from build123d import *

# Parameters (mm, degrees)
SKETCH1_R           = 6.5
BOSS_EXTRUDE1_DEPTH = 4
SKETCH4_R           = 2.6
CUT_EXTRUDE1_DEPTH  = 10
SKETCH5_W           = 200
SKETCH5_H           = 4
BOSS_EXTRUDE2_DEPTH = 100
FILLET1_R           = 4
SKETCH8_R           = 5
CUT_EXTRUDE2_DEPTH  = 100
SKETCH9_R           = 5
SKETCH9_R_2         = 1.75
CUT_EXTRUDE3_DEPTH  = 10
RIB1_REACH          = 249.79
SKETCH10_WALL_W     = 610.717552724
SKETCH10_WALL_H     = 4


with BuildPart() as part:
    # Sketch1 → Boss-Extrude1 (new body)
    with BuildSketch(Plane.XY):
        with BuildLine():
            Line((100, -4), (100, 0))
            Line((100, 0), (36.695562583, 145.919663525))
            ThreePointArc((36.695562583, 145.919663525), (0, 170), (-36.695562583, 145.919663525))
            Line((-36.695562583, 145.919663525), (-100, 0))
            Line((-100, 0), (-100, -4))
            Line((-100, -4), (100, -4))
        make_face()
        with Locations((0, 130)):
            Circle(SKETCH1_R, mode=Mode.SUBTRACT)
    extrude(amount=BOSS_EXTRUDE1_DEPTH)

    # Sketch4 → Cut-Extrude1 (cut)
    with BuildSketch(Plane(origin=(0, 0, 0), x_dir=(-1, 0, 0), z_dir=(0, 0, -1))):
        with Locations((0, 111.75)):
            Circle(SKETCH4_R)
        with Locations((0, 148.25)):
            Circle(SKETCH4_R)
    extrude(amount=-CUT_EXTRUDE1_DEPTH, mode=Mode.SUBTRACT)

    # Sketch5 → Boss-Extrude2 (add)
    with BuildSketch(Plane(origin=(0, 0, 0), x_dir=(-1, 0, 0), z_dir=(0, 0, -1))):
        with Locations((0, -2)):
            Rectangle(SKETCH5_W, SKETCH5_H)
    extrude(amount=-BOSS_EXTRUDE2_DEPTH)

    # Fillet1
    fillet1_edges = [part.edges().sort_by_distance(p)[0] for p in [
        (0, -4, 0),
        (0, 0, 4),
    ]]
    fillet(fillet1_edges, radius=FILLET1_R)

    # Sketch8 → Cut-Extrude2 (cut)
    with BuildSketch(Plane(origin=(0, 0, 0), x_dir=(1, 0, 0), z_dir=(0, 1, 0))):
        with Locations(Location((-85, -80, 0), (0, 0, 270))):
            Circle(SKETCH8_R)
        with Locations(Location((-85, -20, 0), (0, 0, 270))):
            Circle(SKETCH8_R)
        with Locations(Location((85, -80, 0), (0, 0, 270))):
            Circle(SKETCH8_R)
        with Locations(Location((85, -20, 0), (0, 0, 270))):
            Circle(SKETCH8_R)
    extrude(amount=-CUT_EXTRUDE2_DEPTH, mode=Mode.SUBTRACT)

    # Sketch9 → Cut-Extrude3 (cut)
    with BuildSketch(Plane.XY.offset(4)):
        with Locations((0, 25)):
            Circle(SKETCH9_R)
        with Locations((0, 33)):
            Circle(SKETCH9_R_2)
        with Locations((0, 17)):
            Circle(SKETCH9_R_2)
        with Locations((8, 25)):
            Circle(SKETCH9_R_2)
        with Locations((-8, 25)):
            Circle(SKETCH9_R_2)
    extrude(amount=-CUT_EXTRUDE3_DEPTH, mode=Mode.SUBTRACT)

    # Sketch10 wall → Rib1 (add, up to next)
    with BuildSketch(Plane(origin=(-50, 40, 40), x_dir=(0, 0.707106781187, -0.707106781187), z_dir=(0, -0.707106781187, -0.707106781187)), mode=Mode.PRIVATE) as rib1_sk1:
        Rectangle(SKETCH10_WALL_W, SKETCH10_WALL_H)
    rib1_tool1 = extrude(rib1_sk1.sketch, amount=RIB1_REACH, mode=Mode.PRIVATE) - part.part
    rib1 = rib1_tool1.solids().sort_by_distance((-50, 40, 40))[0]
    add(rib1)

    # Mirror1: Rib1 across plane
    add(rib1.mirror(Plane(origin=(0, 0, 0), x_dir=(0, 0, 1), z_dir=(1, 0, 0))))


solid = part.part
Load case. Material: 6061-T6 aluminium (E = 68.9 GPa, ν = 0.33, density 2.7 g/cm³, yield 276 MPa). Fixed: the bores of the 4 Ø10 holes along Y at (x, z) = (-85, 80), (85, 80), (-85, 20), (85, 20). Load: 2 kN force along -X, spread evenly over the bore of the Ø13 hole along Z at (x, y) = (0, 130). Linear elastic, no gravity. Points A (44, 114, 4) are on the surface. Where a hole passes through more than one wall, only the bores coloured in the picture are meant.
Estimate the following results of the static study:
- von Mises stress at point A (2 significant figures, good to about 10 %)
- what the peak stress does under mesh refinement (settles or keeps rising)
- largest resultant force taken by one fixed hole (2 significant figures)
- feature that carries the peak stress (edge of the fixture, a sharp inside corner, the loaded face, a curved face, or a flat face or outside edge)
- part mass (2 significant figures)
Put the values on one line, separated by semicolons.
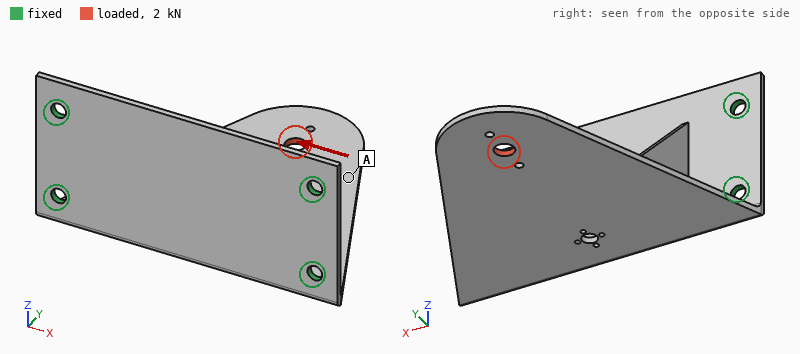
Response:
8.8 MPa; keeps rising; 1.9 kN; edge of the fixture; 500 g
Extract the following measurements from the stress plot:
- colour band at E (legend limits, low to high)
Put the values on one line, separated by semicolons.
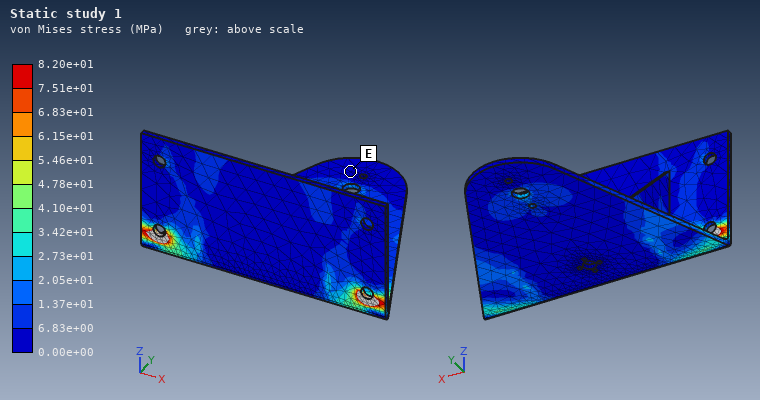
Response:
0.00e+00 to 6.83e+00 MPa
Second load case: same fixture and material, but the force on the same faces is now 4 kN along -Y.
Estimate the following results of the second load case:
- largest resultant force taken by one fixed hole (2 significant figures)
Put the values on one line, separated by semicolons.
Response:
2.5 kN
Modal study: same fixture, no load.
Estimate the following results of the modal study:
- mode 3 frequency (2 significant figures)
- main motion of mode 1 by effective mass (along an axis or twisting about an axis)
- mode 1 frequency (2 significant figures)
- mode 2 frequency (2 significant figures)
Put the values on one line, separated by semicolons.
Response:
1000 Hz; along Z; 330 Hz; 820 Hz
